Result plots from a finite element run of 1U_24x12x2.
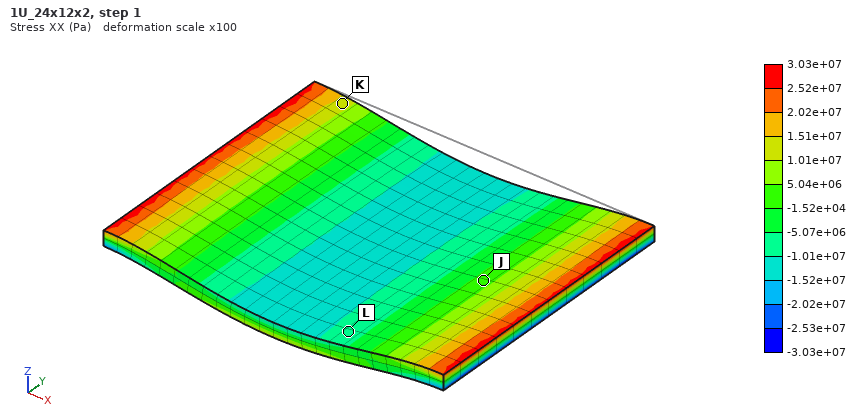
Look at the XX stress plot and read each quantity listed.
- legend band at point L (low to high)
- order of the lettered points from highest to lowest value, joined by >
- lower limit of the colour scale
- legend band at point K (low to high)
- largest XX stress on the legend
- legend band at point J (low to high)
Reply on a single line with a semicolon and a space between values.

-1.01e+07 to -5.07e+06 Pa; K > J > L; -3.03e+07 Pa; 1.01e+07 to 1.51e+07 Pa; 3.03e+07 Pa; -1.52e+04 to 5.04e+06 Pa
